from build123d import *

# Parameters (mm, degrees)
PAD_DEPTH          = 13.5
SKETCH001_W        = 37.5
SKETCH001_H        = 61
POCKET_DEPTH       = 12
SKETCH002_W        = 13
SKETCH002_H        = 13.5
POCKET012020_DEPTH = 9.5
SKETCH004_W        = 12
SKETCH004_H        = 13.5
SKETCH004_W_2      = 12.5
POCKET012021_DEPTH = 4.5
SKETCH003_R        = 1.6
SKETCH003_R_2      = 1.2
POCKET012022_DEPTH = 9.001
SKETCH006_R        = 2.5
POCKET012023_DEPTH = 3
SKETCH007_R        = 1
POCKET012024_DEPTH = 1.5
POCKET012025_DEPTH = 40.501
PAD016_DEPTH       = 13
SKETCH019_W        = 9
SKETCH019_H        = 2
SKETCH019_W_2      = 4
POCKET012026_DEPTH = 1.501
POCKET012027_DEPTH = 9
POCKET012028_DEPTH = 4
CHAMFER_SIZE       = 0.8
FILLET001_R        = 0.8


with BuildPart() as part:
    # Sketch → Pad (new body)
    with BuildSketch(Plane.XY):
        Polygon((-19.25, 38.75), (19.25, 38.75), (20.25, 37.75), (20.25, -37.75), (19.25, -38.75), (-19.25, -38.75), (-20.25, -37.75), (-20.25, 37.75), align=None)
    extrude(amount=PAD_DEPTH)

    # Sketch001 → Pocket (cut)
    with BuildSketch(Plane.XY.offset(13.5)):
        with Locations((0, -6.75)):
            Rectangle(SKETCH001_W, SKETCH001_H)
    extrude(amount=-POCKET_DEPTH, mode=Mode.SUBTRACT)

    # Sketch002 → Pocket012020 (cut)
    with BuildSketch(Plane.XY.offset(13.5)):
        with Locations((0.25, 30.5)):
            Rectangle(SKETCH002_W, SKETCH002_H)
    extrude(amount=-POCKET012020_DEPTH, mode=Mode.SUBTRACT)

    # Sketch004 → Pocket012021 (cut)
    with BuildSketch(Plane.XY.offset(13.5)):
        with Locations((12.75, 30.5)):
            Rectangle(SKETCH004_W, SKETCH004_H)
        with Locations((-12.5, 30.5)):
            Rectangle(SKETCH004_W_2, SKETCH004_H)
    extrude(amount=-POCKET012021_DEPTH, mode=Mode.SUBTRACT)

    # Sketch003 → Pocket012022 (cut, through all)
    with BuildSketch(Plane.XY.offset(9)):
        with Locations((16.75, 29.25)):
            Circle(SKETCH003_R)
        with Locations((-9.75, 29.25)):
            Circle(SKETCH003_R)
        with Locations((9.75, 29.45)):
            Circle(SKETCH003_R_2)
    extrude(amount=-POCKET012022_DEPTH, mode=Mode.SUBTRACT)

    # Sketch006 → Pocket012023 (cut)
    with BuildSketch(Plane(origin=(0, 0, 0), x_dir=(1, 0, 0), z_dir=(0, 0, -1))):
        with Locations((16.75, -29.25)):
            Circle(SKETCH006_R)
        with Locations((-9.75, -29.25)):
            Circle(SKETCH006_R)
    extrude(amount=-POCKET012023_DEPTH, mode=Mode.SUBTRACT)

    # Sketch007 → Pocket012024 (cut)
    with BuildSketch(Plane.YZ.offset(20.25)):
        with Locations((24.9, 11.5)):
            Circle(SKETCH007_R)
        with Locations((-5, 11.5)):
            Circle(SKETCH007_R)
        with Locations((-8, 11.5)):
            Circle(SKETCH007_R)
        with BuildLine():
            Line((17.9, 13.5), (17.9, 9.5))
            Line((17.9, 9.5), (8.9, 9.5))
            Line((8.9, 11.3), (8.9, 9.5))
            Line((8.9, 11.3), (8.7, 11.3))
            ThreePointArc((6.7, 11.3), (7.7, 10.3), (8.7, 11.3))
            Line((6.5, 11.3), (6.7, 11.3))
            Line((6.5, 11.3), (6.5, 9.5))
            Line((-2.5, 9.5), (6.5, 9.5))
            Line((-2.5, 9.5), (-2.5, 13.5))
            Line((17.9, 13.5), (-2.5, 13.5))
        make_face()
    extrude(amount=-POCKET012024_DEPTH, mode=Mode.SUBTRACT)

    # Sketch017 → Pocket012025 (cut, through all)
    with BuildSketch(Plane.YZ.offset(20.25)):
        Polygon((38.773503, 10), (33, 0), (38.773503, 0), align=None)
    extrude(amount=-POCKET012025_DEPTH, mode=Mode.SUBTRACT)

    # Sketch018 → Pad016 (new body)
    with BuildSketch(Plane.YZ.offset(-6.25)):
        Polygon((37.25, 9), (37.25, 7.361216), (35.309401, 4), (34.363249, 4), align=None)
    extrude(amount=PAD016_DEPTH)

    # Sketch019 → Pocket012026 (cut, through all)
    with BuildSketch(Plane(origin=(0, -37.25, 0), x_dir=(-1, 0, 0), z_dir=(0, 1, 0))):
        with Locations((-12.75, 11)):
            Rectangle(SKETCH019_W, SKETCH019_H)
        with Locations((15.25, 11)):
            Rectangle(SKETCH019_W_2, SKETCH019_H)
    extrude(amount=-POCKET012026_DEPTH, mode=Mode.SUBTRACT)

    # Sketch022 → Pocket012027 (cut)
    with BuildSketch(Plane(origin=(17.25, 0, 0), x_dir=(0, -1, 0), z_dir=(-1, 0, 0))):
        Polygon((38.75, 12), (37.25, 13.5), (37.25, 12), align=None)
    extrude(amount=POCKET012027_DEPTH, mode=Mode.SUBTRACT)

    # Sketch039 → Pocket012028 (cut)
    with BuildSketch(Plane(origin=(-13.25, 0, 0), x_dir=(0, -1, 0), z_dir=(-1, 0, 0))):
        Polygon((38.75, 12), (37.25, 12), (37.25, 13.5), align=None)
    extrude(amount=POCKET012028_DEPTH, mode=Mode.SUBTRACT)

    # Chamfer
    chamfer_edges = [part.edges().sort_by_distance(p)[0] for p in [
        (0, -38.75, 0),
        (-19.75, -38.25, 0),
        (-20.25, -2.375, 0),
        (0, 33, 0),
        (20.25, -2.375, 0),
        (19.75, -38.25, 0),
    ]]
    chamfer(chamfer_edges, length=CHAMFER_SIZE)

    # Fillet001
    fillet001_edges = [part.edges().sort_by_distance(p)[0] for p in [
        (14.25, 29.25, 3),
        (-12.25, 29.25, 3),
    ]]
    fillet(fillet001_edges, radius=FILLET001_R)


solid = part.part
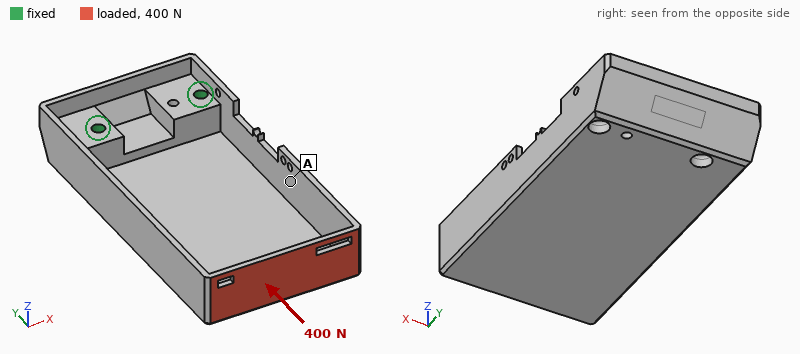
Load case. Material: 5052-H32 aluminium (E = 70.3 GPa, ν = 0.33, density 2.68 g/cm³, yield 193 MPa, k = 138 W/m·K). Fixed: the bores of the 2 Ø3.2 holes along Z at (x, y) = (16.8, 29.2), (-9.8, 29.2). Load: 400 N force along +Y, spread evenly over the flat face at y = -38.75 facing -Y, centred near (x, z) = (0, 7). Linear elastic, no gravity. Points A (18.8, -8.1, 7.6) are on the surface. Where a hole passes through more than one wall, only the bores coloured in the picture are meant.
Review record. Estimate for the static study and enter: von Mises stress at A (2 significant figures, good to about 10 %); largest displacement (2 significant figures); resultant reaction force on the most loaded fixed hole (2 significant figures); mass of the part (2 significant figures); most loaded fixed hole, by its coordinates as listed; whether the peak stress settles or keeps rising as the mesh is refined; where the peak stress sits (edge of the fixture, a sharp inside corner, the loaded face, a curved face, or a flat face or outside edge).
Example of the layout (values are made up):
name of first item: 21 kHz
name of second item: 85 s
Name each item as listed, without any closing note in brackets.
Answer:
von Mises stress at A: 12 MPa
largest displacement: 0.20 mm
resultant reaction force on the most loaded fixed hole: 240 N
mass of the part: 27 g
most loaded fixed hole, by its coordinates as listed: (-9.8, 29.2)
whether the peak stress settles or keeps rising as the mesh is refined: keeps rising
where the peak stress sits: a sharp inside corner
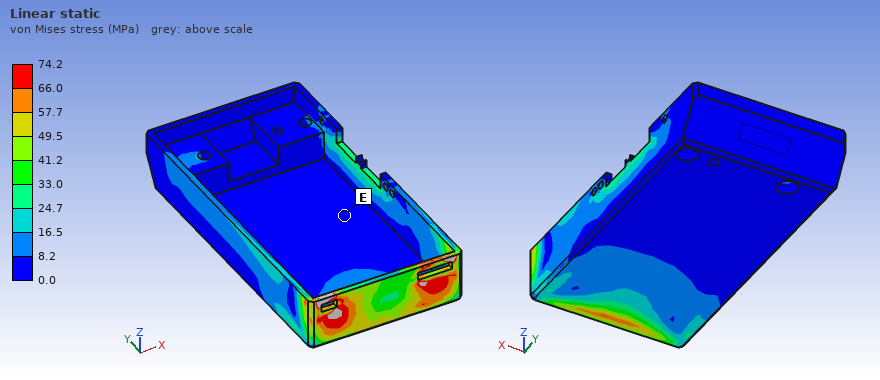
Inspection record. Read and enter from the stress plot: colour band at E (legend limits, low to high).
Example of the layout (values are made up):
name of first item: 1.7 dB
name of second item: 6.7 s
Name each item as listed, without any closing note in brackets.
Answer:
colour band at E: 0.0 to 8.2 MPa
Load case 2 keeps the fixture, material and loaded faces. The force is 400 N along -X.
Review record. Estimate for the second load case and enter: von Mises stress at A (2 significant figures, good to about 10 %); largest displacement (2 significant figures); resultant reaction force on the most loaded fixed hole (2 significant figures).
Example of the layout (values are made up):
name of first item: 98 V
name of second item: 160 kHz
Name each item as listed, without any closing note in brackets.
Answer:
von Mises stress at A: 27 MPa
largest displacement: 0.62 mm
resultant reaction force on the most loaded fixed hole: 950 N
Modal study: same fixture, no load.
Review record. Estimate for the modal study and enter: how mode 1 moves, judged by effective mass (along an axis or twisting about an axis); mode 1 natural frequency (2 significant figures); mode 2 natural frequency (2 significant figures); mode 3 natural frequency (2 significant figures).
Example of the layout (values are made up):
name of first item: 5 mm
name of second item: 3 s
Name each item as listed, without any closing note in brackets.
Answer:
how mode 1 moves, judged by effective mass: along Z
mode 1 natural frequency: 1300 Hz
mode 2 natural frequency: 1700 Hz
mode 3 natural frequency: 4000 Hz
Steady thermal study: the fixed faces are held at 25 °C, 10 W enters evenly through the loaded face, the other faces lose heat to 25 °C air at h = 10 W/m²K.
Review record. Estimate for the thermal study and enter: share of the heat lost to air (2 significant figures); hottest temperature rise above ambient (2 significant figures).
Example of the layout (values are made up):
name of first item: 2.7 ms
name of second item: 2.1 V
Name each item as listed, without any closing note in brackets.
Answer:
share of the heat lost to air: 21 %
hottest temperature rise above ambient: 51 K
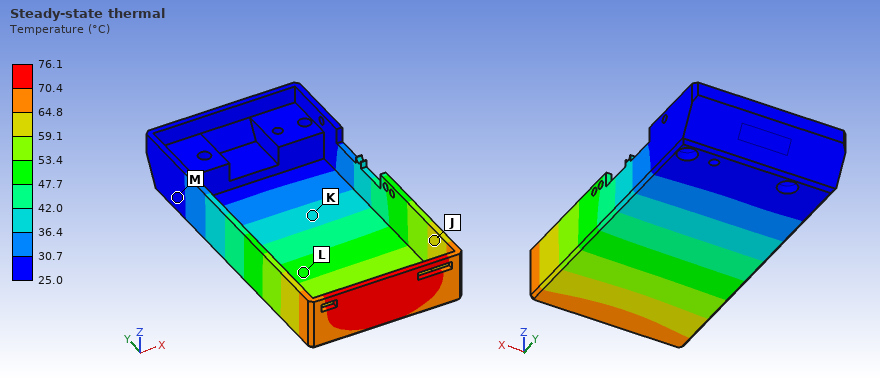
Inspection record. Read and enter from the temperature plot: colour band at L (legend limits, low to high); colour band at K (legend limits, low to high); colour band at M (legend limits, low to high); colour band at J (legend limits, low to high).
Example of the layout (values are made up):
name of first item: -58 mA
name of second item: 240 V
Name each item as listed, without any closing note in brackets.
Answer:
colour band at L: 47.7 to 53.4 °C
colour band at K: 36.4 to 42.0 °C
colour band at M: 25.0 to 30.7 °C
colour band at J: 59.1 to 64.8 °C
